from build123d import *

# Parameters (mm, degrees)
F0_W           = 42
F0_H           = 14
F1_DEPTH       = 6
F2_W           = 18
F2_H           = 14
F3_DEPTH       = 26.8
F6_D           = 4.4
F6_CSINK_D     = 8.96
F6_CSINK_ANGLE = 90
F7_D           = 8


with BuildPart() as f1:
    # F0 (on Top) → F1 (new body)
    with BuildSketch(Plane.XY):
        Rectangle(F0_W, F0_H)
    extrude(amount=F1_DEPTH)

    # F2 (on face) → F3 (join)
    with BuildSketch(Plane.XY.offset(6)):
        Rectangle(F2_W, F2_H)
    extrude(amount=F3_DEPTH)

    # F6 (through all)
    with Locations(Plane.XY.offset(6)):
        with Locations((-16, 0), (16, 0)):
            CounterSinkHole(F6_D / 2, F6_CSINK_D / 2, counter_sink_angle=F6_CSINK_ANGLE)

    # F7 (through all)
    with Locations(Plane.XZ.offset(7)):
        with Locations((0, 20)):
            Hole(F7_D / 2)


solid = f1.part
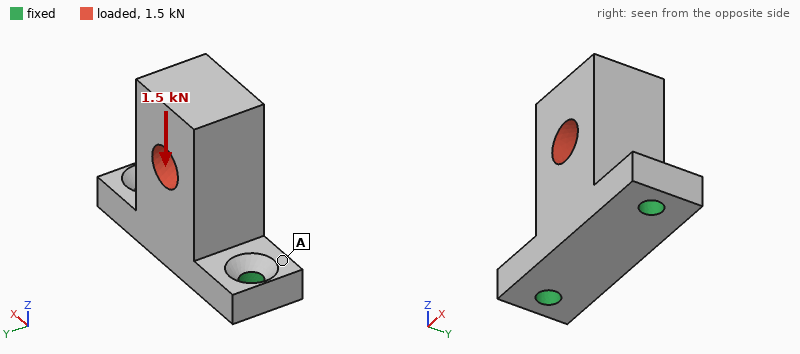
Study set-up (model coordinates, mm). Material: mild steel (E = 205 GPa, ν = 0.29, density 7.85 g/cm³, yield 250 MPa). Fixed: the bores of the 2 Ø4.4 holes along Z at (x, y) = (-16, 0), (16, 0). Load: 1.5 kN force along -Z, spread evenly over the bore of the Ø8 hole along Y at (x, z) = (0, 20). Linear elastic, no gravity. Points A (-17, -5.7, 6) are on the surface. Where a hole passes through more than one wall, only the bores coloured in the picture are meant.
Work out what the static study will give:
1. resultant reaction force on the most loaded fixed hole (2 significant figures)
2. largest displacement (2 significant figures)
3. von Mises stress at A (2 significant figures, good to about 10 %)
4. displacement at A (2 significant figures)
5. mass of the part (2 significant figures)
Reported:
890 N
3.3 µm
10 MPa
0.57 µm
73 g
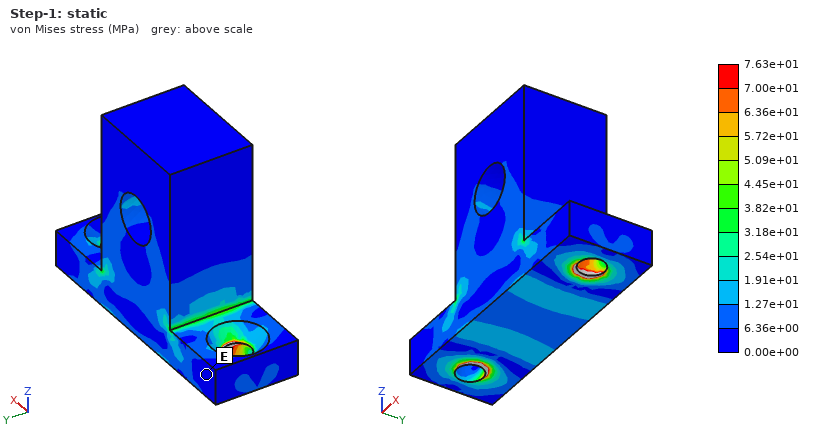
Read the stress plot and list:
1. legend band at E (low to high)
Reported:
0.00e+00 to 6.36e+00 MPa
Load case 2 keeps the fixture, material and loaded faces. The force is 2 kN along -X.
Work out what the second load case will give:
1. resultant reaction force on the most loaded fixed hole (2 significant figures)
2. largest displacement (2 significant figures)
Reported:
1.7 kN
17 µm
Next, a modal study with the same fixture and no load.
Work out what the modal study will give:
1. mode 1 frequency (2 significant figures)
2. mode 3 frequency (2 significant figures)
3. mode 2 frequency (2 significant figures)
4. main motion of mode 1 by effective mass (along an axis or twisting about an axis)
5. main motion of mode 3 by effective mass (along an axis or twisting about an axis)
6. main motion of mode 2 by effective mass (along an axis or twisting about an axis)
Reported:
3800 Hz
15 kHz
9200 Hz
along Y
along Z
along X
